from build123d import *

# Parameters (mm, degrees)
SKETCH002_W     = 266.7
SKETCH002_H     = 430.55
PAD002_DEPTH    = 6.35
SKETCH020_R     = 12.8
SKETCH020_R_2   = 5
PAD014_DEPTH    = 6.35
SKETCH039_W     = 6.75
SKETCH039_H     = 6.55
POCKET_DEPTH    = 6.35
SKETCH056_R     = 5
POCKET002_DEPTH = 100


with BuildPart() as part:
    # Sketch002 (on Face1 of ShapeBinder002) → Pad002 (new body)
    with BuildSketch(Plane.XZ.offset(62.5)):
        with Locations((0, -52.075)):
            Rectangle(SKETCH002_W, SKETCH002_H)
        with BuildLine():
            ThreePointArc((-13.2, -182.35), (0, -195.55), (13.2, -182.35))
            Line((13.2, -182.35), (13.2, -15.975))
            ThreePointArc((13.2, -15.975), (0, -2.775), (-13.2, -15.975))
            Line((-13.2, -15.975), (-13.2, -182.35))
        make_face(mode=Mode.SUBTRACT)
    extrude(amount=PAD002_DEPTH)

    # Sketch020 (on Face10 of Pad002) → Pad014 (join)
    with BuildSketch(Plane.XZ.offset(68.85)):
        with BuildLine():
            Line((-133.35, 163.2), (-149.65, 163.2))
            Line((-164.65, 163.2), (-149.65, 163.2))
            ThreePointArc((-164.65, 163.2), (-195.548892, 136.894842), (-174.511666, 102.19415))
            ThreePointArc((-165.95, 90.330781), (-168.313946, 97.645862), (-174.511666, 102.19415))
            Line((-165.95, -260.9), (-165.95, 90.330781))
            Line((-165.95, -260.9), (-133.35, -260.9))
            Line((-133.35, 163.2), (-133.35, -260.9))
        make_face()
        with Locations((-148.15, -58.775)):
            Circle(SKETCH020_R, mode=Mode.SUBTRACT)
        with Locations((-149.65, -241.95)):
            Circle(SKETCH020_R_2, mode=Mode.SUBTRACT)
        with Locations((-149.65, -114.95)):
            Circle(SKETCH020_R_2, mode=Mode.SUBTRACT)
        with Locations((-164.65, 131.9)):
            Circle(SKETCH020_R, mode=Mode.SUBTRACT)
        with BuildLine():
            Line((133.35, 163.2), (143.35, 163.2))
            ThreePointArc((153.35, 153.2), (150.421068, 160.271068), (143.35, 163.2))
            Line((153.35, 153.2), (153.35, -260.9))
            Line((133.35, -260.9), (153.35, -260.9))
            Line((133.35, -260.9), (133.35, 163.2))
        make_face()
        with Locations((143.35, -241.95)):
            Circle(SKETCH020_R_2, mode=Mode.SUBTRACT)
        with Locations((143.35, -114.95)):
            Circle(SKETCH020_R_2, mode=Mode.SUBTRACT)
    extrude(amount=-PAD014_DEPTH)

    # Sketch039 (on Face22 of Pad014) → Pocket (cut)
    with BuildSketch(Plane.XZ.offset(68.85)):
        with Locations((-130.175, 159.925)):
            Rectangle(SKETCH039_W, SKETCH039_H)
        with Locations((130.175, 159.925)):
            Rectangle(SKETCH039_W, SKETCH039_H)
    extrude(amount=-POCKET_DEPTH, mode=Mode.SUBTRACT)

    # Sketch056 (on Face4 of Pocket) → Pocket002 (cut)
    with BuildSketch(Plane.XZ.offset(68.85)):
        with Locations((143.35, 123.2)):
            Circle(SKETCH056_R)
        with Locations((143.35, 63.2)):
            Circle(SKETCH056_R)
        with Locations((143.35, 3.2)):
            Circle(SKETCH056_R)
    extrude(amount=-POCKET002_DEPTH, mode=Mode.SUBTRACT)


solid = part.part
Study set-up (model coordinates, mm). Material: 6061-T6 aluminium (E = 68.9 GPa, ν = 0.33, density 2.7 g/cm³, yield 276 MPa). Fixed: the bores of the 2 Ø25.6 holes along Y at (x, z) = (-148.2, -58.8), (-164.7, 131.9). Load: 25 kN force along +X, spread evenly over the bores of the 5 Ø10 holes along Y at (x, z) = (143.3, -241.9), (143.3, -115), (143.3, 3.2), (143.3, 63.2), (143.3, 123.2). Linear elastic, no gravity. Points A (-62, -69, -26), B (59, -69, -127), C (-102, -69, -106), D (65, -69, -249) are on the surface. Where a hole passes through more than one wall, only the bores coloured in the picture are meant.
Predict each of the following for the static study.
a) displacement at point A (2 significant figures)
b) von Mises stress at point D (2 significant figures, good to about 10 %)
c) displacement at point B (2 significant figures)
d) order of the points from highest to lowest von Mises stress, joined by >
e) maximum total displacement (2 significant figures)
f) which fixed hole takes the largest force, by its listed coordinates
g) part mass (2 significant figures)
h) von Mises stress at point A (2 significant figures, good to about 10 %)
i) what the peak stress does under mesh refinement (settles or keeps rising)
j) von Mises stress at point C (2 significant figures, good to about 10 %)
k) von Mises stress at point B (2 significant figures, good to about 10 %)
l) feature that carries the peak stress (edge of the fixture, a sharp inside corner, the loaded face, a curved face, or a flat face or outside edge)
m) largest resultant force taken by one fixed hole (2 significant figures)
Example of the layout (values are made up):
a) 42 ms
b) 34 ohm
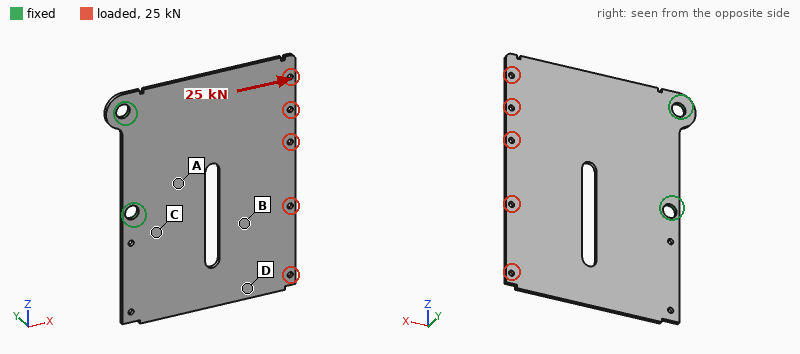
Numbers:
a) 0.049 mm
b) 14 MPa
c) 0.22 mm
d) A > C > D > B
e) 0.30 mm
f) (-148.2, -58.8)
g) 2.3 kg
h) 32 MPa
i) keeps rising
j) 22 MPa
k) 6.3 MPa
l) edge of the fixture
m) 21 kN
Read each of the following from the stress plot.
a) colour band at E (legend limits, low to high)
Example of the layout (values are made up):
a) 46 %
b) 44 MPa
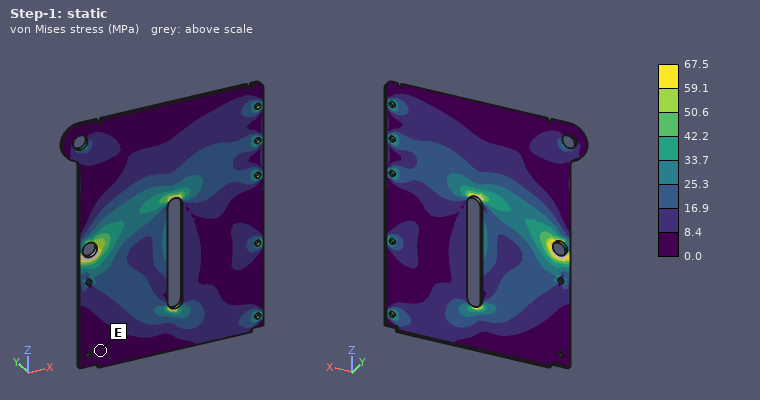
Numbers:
a) 0.0 to 8.4 MPa
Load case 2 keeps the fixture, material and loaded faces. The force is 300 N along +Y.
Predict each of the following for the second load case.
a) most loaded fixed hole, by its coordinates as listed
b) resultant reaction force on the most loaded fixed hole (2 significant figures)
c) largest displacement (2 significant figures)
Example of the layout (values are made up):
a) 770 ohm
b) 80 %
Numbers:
a) (-148.2, -58.8)
b) 290 N
c) 6.6 mm
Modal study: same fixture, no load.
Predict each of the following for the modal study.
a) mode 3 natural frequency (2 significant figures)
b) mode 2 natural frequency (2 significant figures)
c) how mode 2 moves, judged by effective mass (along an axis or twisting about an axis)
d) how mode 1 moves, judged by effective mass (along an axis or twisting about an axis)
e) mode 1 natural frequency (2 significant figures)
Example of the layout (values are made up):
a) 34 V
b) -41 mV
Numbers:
a) 160 Hz
b) 76 Hz
c) twisting about X
d) along Y
e) 45 Hz
